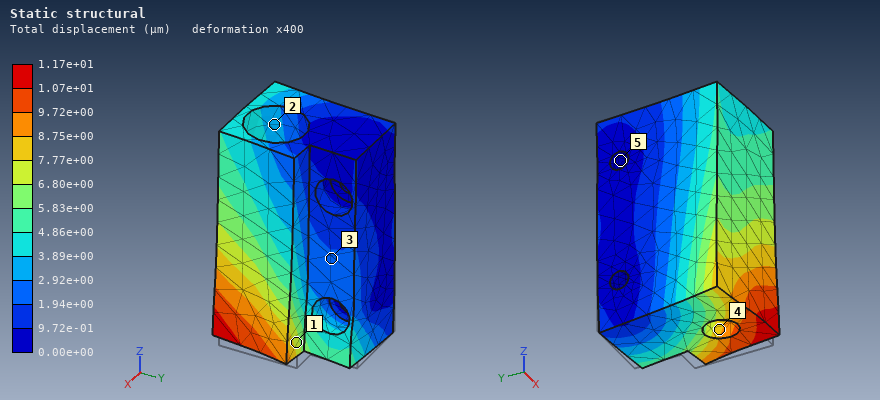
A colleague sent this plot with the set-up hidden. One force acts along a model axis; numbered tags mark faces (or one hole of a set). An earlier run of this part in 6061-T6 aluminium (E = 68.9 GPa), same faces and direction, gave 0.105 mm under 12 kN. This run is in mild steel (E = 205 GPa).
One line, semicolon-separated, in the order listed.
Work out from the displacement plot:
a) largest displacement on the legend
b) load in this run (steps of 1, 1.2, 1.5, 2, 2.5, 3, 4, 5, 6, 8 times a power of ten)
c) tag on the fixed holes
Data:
1.17e+01 µm; 4 kN; 5
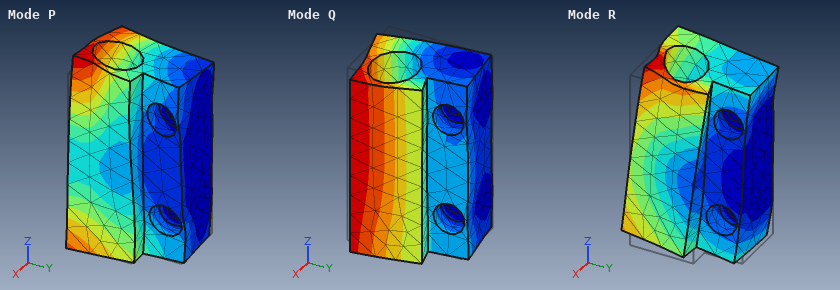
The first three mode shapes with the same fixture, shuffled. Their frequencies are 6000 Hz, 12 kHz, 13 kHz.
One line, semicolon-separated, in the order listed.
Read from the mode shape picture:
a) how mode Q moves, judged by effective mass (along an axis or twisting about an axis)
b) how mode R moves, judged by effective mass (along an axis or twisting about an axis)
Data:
along X; along Z
